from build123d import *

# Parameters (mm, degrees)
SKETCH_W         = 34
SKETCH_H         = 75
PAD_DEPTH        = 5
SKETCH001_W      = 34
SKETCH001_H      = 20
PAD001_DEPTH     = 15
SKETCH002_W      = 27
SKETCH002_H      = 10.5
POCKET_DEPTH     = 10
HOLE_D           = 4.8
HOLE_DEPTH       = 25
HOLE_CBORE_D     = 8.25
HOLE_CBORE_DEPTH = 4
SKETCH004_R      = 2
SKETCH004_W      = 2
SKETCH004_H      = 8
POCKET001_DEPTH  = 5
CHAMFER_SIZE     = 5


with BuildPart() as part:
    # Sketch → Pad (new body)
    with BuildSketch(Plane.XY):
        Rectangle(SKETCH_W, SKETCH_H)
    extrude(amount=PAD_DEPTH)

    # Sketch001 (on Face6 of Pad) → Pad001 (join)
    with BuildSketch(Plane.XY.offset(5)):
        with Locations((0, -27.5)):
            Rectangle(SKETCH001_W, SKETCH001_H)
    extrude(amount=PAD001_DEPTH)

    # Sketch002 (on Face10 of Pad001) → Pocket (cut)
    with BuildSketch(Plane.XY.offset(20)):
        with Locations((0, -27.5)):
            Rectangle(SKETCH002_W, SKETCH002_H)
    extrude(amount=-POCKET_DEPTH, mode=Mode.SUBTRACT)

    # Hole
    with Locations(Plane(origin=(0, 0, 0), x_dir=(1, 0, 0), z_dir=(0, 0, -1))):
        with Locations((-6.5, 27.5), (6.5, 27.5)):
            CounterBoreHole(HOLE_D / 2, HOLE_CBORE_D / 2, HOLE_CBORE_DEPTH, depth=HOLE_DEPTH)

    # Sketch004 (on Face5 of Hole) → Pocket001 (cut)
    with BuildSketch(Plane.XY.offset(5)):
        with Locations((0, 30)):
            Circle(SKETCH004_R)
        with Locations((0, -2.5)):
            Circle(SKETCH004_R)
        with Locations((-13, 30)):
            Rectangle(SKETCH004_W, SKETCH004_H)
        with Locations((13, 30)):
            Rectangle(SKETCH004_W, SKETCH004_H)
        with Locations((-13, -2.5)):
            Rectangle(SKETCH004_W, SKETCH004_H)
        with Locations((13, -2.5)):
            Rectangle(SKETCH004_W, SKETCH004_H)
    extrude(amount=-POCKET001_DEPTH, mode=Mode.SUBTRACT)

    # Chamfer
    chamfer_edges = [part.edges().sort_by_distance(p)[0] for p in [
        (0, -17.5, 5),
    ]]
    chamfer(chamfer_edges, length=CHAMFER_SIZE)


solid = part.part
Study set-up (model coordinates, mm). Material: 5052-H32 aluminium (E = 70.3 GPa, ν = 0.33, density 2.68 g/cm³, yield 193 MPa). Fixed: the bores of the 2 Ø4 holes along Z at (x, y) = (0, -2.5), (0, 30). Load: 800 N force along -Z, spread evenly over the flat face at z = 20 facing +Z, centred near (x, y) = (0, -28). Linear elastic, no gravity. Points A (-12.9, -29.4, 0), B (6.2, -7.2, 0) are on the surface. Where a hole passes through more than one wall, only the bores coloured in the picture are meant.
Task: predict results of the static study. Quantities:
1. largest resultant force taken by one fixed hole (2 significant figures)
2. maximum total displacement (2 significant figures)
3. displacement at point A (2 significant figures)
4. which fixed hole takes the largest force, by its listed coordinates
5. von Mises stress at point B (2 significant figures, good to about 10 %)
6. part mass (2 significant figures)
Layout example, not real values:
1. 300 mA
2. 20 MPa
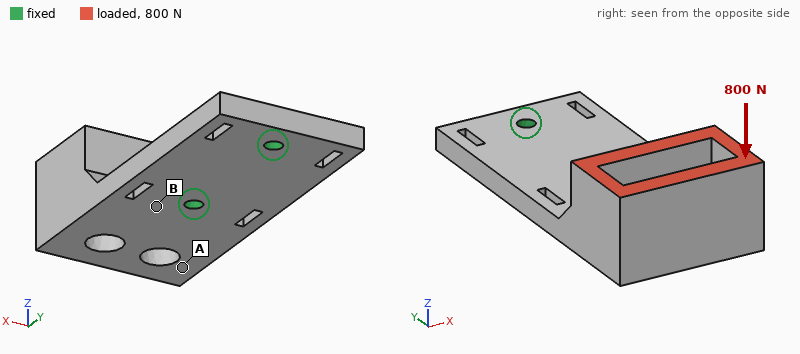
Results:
1. 1.0 kN
2. 0.32 mm
3. 0.21 mm
4. (0, -2.5)
5. 100 MPa
6. 52 g
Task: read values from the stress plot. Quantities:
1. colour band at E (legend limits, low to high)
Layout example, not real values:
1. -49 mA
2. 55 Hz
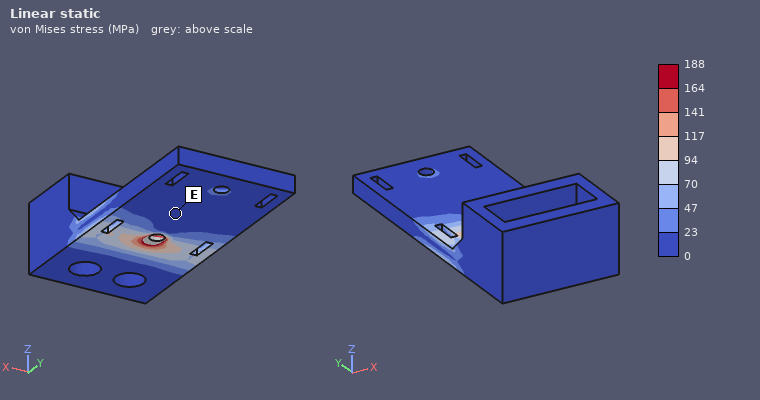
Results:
1. 0 to 23 MPa
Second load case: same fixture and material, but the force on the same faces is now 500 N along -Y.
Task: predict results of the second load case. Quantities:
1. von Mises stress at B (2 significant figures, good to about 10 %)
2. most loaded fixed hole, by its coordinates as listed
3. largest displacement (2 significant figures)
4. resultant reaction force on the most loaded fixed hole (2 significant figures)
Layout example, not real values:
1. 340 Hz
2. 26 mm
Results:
1. 54 MPa
2. (0, -2.5)
3. 0.18 mm
4. 420 N
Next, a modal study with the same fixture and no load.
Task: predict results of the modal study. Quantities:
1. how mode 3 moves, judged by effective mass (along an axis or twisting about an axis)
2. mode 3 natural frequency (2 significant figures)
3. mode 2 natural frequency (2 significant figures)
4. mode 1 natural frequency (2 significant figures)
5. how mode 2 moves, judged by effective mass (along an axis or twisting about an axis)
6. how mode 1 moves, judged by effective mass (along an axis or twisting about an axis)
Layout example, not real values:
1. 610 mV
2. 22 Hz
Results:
1. along X
2. 6200 Hz
3. 3400 Hz
4. 1700 Hz
5. along X
6. along Z
